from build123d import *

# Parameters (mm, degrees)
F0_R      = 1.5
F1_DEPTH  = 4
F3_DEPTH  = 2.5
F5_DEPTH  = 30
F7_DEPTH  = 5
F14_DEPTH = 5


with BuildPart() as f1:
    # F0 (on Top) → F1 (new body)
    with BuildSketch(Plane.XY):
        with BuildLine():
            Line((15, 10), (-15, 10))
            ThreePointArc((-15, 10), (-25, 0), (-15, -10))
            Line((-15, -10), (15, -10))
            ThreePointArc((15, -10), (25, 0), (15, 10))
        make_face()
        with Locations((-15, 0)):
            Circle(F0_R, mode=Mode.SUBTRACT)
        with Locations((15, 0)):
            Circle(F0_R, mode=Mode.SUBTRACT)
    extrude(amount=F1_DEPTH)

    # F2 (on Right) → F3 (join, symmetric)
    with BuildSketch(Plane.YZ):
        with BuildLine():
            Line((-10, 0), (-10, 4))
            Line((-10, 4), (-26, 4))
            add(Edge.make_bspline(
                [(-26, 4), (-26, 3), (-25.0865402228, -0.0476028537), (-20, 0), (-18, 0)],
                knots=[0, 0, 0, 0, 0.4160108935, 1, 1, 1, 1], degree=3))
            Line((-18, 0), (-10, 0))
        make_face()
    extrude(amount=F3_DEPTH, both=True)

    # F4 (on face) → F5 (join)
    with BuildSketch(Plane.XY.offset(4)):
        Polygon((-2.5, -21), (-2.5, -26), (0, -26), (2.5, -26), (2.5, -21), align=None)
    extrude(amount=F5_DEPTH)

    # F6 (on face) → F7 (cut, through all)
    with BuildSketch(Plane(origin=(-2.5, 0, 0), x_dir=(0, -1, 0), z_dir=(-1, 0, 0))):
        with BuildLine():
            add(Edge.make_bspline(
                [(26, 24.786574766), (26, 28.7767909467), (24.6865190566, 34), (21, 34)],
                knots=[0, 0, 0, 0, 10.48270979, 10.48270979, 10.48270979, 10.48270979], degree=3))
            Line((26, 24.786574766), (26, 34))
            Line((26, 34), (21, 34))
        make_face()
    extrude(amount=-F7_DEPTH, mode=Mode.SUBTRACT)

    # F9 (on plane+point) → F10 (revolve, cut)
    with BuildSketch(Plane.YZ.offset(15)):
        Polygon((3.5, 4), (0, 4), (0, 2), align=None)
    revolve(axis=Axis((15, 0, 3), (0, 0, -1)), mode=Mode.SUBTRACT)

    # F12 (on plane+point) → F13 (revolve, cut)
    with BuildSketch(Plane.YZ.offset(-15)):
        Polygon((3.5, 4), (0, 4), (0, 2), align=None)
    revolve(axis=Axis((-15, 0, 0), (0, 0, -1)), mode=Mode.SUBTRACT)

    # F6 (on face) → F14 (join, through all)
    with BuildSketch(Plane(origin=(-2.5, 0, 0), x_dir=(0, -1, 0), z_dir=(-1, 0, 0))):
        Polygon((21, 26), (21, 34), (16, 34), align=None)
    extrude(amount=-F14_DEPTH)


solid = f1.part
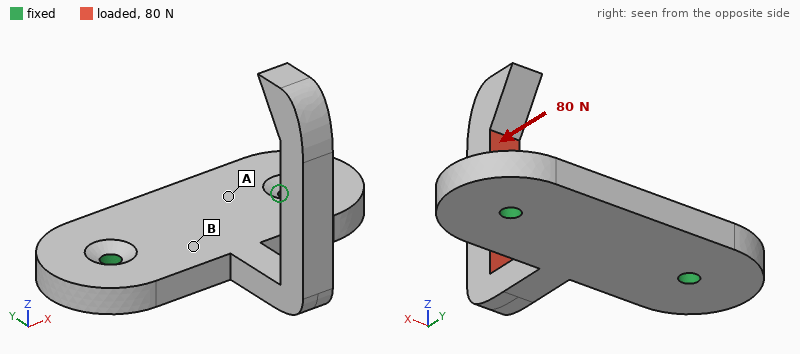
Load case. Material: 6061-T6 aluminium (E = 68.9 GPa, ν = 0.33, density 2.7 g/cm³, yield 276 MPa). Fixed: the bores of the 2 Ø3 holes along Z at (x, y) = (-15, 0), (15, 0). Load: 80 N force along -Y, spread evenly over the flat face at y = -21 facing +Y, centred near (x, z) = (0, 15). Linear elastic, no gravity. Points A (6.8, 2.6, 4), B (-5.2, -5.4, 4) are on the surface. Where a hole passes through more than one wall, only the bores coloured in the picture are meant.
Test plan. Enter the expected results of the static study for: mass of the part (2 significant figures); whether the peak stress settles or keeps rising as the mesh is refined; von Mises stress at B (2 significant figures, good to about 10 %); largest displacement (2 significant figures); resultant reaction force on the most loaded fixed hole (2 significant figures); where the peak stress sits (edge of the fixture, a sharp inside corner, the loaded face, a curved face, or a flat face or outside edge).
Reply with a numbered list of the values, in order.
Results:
1. 13 g
2. keeps rising
3. 21 MPa
4. 0.38 mm
5. 40 N
6. a sharp inside corner
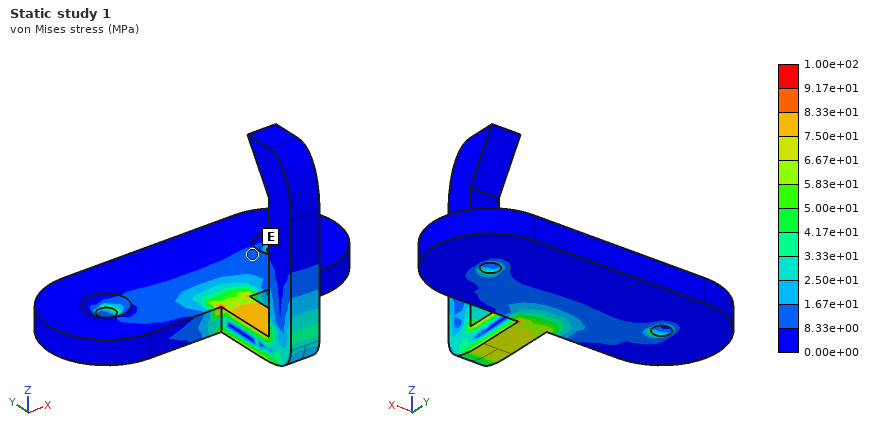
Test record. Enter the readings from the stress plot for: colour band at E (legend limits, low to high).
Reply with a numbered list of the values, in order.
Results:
1. 8.33e+00 to 1.67e+01 MPa
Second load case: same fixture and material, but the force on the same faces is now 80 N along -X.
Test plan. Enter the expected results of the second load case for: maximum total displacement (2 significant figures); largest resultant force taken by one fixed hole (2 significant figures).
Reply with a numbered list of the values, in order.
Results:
1. 0.41 mm
2. 82 N
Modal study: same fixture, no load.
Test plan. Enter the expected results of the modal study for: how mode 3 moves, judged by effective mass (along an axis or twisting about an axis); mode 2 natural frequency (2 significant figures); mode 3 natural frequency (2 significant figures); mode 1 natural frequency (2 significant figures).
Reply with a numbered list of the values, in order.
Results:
1. along Z
2. 1500 Hz
3. 4300 Hz
4. 1400 Hz
